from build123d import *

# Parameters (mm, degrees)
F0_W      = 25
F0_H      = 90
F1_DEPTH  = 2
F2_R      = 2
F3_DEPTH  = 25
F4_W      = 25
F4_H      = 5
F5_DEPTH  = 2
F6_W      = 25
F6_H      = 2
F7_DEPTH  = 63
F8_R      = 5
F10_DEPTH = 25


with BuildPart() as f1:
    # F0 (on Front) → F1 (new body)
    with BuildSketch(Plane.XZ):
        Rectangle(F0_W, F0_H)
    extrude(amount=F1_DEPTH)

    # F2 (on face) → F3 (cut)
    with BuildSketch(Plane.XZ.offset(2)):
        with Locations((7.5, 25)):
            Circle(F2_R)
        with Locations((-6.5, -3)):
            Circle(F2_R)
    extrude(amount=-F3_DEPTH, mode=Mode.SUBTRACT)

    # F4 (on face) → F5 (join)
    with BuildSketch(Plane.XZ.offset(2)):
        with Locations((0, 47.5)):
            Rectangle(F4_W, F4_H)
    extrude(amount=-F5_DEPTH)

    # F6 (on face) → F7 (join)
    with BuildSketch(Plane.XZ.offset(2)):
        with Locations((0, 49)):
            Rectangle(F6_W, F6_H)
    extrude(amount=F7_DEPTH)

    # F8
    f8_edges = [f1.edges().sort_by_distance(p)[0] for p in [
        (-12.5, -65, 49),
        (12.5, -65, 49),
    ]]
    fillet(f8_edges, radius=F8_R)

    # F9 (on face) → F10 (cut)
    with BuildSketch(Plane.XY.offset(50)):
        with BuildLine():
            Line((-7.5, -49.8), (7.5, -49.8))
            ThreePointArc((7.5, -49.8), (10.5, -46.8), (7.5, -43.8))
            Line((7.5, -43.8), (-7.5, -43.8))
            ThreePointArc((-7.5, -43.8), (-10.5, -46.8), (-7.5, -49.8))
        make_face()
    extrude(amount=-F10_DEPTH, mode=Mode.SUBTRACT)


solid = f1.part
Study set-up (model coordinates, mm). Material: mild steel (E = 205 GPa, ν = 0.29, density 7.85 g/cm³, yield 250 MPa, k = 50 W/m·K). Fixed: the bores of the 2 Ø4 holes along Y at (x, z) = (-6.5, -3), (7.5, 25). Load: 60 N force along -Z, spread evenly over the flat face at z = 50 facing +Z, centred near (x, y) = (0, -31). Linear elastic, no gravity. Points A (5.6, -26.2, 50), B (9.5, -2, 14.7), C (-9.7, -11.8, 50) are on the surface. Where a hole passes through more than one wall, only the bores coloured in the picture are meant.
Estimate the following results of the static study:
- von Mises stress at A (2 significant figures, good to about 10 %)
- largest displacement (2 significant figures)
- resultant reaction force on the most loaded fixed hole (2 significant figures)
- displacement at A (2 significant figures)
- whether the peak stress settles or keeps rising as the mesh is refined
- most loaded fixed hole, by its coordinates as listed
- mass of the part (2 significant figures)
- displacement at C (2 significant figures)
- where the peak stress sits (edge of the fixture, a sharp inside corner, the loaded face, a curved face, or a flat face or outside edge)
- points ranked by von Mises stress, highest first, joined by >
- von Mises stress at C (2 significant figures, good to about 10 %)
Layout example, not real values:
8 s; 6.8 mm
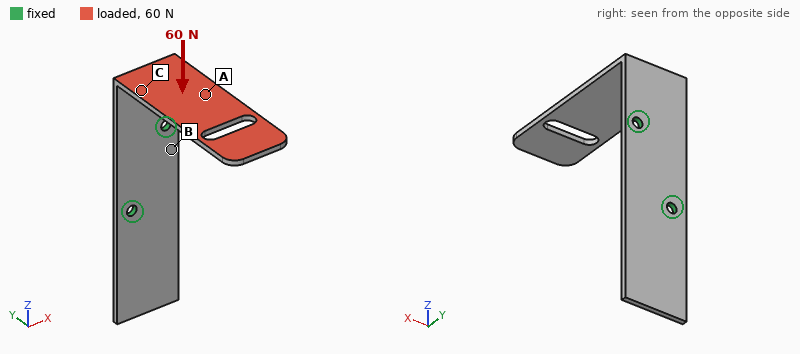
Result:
38 MPa; 1.4 mm; 48 N; 0.47 mm; keeps rising; (7.5, 25); 60 g; 0.24 mm; edge of the fixture; C > A > B; 74 MPa
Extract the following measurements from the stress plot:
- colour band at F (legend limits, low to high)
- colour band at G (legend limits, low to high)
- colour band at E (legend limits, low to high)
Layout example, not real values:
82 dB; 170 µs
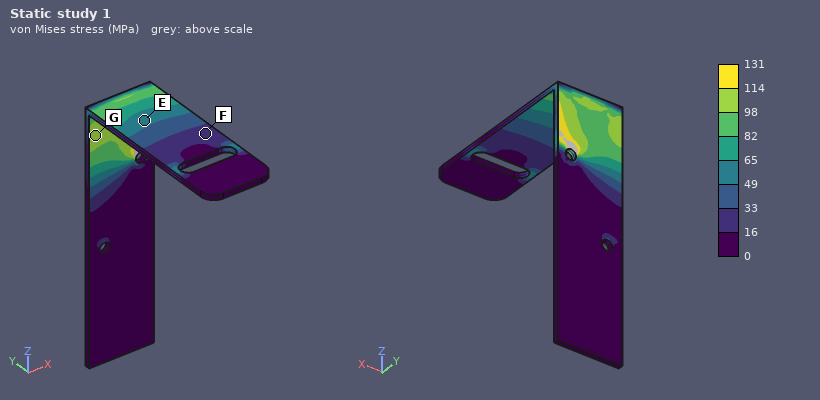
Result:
16 to 33 MPa; 98 to 114 MPa; 49 to 65 MPa
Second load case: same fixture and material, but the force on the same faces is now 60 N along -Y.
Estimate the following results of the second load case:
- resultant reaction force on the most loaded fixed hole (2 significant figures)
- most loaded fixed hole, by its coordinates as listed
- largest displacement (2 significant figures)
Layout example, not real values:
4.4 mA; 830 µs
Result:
76 N; (7.5, 25); 0.42 mm
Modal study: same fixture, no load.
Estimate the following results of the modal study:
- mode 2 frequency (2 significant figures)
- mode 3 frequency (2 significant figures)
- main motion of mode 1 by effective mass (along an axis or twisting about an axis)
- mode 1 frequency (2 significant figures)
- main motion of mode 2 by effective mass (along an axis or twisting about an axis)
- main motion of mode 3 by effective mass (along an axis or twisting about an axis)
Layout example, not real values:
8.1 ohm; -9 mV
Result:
430 Hz; 910 Hz; along Z; 270 Hz; along X; along Y
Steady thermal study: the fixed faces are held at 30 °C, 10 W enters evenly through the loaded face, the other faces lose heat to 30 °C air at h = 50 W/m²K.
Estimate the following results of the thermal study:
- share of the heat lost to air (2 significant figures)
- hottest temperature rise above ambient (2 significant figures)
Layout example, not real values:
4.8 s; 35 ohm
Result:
73 %; 79 K
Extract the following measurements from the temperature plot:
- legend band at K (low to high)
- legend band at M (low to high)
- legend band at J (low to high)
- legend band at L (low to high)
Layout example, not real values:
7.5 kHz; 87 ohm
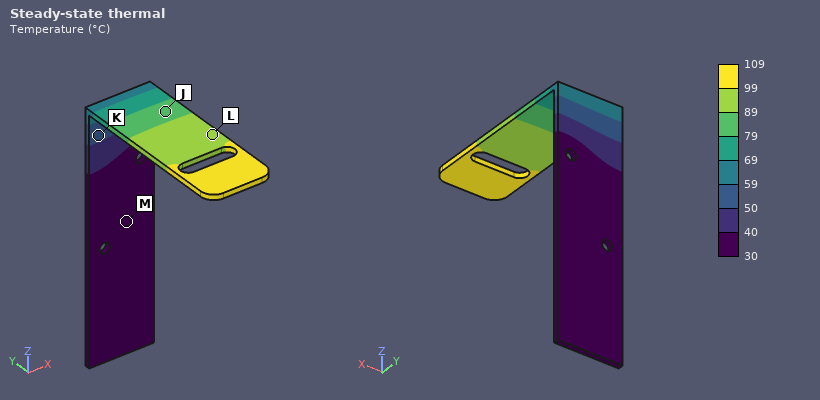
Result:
50 to 59 °C; 30 to 40 °C; 79 to 89 °C; 89 to 99 °C
